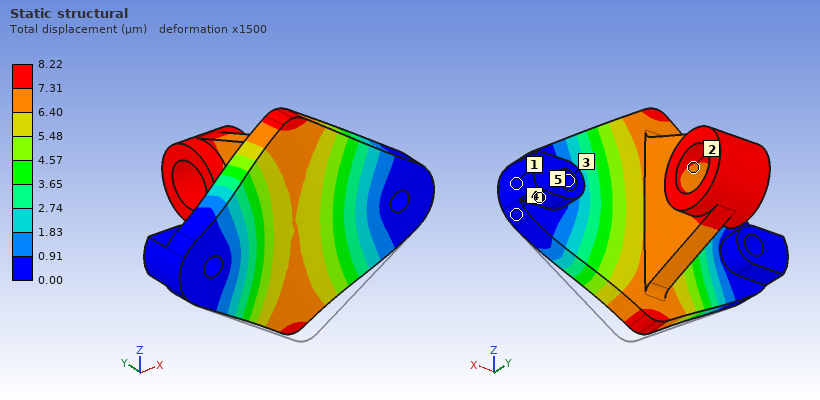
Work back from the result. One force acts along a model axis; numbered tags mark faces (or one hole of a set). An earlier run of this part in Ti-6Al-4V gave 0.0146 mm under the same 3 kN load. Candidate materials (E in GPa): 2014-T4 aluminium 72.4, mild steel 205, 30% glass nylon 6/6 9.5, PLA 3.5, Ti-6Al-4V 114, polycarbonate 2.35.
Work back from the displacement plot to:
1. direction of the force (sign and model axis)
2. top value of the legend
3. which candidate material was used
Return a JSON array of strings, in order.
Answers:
["+Y", "8.22 µm", "mild steel"]
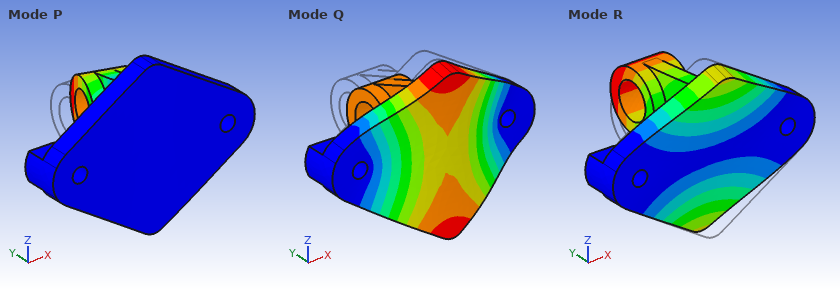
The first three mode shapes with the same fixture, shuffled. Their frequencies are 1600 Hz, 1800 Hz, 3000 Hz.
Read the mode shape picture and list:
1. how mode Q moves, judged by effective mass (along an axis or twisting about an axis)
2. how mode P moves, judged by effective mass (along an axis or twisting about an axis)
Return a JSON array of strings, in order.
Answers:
["along Y", "along X"]
